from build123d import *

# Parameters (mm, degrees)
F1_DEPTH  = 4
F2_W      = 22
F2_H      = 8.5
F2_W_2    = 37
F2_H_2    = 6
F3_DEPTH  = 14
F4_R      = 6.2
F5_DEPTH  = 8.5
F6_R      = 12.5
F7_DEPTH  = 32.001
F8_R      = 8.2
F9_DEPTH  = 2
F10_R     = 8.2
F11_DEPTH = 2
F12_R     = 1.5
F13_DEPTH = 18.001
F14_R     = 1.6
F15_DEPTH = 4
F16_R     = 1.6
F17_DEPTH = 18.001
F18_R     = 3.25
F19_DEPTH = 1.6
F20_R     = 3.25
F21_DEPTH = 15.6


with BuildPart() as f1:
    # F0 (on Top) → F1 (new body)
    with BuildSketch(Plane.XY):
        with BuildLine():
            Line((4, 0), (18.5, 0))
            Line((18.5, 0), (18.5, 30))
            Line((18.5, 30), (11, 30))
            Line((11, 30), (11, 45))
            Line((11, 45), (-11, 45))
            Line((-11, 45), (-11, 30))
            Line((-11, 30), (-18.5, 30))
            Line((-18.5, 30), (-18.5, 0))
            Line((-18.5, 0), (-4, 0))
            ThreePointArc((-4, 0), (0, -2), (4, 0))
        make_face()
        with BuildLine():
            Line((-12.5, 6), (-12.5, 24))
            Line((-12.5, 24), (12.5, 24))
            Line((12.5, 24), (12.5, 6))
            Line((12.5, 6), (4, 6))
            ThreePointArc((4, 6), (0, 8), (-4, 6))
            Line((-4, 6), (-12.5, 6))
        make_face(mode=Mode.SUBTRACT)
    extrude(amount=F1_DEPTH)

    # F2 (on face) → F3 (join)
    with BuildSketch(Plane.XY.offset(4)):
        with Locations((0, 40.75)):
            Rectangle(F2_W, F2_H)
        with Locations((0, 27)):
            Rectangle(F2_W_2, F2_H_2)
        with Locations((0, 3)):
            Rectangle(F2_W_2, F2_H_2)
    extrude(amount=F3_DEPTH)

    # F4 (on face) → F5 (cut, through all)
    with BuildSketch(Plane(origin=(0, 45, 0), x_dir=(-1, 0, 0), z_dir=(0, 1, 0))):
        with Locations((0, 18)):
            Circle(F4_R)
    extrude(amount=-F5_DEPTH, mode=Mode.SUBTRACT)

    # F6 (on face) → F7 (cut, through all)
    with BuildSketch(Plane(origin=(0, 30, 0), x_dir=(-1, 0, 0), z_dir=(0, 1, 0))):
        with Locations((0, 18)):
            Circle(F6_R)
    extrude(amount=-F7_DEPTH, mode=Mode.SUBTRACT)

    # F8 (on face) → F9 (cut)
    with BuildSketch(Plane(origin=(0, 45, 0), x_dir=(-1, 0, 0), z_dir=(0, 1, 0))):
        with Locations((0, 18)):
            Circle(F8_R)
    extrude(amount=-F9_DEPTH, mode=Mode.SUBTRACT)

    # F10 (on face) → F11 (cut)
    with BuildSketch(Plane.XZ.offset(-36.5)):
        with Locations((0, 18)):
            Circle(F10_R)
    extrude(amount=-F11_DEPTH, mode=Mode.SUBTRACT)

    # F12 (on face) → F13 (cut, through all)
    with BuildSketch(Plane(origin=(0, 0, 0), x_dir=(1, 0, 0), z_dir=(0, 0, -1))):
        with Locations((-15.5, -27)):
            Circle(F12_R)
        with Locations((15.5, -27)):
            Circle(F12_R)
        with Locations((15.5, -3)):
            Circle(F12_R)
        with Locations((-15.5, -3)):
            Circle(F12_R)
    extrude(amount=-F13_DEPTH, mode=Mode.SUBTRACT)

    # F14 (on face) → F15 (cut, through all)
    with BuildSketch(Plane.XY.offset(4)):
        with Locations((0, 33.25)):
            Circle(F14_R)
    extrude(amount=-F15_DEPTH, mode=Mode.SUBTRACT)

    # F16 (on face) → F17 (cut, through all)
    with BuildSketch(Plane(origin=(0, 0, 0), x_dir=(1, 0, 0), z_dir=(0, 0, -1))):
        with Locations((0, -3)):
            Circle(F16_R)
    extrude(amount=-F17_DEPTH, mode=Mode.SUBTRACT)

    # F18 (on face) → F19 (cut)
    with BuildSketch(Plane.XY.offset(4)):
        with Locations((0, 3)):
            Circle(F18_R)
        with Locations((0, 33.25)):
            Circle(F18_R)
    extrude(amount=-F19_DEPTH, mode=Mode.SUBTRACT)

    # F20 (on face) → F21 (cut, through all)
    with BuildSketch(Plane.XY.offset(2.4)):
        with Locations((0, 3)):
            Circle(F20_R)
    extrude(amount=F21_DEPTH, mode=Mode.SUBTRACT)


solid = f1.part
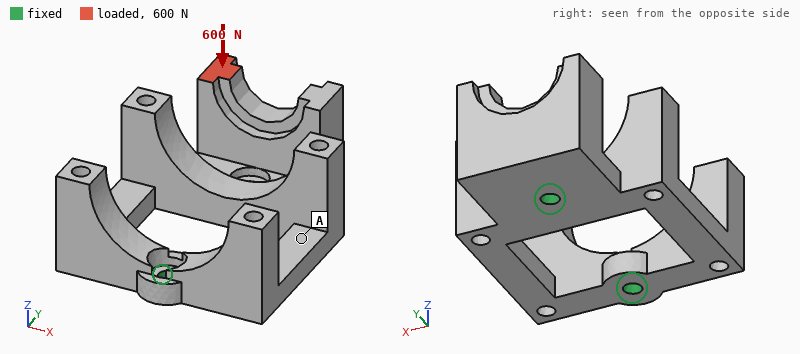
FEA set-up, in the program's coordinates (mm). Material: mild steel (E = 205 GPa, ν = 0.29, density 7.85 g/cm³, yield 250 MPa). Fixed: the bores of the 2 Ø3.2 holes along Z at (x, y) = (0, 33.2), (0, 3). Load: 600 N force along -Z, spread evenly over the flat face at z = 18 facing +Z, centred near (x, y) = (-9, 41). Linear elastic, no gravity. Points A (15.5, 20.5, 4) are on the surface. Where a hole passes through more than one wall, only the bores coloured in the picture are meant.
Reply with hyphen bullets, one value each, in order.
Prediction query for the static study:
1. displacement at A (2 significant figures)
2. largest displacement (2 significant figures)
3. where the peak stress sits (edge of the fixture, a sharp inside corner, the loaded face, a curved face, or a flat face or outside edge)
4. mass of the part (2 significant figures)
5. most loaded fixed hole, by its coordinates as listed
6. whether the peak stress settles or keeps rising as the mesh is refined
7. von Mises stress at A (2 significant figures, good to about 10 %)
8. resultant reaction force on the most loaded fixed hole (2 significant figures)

- 19 µm
- 50 µm
- edge of the fixture
- 67 g
- (0, 33.2)
- keeps rising
- 26 MPa
- 650 N
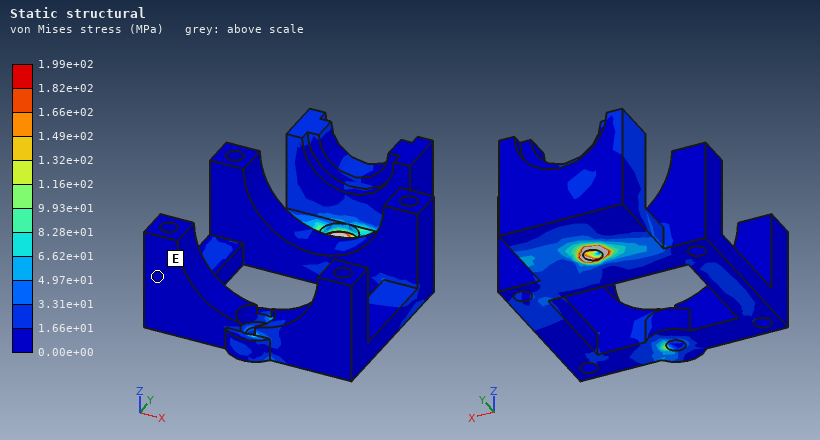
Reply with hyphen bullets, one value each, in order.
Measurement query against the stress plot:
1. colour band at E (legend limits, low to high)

- 0.00e+00 to 1.66e+01 MPa
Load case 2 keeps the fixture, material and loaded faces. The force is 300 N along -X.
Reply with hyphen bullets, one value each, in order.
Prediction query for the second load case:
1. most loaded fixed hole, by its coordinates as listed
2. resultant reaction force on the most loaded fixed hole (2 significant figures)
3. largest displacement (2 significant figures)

- (0, 33.2)
- 330 N
- 34 µm
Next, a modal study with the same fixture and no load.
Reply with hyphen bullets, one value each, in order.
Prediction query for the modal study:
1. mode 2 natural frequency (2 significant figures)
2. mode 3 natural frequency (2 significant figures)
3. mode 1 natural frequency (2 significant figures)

- 4300 Hz
- 5700 Hz
- 3400 Hz
